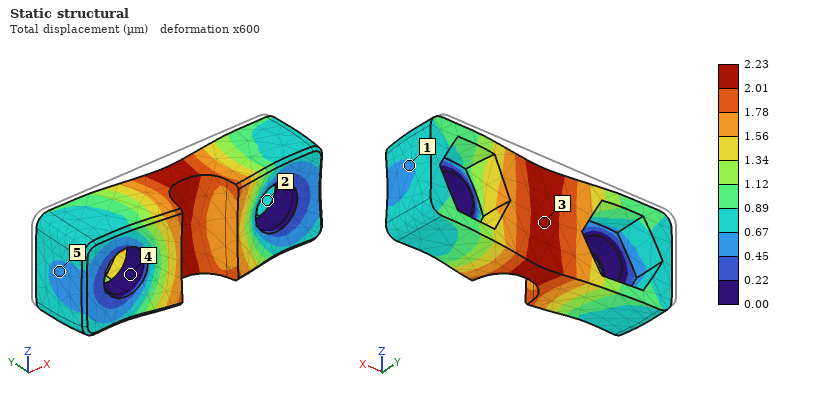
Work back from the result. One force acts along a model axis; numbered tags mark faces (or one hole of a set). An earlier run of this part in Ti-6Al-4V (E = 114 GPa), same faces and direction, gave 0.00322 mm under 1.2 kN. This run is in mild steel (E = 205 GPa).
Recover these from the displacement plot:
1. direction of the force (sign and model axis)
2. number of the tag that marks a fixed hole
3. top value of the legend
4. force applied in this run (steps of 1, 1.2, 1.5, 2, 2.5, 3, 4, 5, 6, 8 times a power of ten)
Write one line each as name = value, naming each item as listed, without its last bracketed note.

direction of the force = -Y
number of the tag that marks a fixed hole = 4
top value of the legend = 2.23 µm
force applied in this run = 1.5 kN
